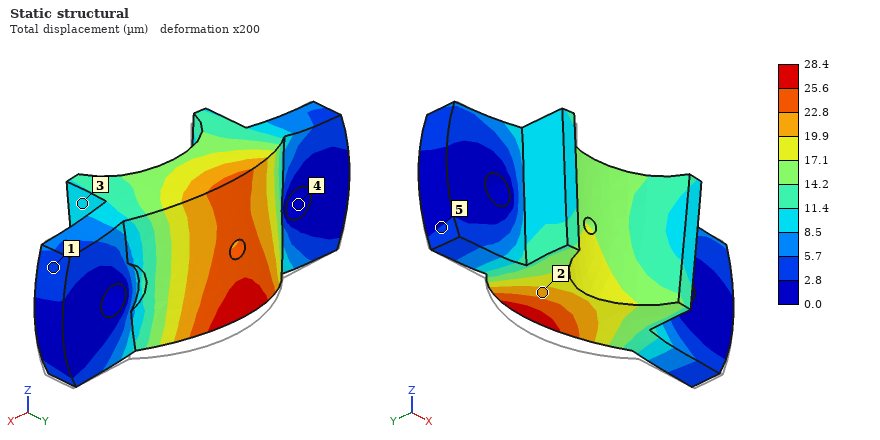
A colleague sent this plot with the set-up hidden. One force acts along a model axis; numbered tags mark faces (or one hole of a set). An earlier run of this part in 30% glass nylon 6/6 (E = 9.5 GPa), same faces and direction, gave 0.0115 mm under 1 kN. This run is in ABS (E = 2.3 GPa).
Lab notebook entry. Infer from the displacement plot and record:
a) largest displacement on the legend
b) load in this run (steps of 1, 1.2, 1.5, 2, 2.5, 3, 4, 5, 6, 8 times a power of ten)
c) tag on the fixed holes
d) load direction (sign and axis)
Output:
28.4 µm
600 N
4
+Z
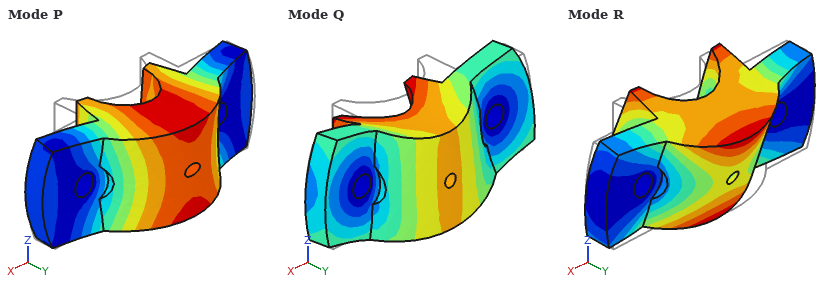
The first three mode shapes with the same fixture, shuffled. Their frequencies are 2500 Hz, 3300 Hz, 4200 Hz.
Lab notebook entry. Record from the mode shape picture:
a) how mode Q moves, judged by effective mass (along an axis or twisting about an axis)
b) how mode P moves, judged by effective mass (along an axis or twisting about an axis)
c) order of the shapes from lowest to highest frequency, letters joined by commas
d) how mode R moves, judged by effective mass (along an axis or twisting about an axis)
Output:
along Z
along Y
R, P, Q
twisting about X
